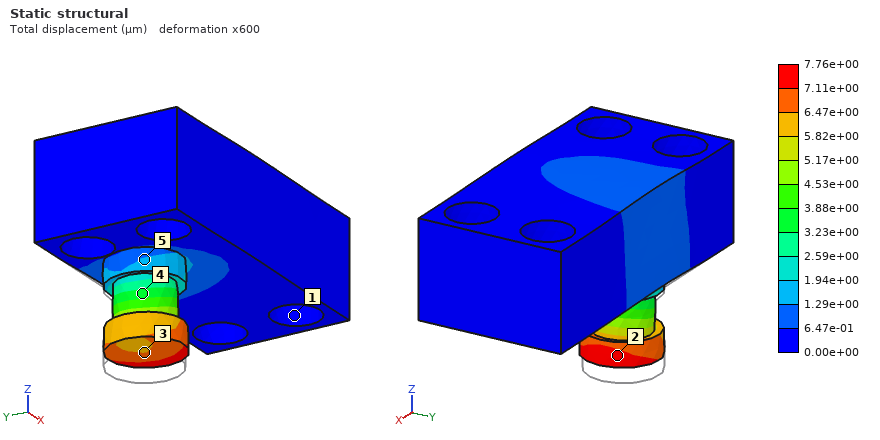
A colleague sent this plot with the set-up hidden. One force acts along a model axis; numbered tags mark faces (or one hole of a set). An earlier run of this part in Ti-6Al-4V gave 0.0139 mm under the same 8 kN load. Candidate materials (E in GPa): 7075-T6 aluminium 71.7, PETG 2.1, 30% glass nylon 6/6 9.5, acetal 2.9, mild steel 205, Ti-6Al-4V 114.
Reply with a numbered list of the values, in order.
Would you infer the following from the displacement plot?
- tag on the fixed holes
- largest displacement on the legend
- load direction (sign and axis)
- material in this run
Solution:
1. 1
2. 7.76e+00 µm
3. +Z
4. mild steel
